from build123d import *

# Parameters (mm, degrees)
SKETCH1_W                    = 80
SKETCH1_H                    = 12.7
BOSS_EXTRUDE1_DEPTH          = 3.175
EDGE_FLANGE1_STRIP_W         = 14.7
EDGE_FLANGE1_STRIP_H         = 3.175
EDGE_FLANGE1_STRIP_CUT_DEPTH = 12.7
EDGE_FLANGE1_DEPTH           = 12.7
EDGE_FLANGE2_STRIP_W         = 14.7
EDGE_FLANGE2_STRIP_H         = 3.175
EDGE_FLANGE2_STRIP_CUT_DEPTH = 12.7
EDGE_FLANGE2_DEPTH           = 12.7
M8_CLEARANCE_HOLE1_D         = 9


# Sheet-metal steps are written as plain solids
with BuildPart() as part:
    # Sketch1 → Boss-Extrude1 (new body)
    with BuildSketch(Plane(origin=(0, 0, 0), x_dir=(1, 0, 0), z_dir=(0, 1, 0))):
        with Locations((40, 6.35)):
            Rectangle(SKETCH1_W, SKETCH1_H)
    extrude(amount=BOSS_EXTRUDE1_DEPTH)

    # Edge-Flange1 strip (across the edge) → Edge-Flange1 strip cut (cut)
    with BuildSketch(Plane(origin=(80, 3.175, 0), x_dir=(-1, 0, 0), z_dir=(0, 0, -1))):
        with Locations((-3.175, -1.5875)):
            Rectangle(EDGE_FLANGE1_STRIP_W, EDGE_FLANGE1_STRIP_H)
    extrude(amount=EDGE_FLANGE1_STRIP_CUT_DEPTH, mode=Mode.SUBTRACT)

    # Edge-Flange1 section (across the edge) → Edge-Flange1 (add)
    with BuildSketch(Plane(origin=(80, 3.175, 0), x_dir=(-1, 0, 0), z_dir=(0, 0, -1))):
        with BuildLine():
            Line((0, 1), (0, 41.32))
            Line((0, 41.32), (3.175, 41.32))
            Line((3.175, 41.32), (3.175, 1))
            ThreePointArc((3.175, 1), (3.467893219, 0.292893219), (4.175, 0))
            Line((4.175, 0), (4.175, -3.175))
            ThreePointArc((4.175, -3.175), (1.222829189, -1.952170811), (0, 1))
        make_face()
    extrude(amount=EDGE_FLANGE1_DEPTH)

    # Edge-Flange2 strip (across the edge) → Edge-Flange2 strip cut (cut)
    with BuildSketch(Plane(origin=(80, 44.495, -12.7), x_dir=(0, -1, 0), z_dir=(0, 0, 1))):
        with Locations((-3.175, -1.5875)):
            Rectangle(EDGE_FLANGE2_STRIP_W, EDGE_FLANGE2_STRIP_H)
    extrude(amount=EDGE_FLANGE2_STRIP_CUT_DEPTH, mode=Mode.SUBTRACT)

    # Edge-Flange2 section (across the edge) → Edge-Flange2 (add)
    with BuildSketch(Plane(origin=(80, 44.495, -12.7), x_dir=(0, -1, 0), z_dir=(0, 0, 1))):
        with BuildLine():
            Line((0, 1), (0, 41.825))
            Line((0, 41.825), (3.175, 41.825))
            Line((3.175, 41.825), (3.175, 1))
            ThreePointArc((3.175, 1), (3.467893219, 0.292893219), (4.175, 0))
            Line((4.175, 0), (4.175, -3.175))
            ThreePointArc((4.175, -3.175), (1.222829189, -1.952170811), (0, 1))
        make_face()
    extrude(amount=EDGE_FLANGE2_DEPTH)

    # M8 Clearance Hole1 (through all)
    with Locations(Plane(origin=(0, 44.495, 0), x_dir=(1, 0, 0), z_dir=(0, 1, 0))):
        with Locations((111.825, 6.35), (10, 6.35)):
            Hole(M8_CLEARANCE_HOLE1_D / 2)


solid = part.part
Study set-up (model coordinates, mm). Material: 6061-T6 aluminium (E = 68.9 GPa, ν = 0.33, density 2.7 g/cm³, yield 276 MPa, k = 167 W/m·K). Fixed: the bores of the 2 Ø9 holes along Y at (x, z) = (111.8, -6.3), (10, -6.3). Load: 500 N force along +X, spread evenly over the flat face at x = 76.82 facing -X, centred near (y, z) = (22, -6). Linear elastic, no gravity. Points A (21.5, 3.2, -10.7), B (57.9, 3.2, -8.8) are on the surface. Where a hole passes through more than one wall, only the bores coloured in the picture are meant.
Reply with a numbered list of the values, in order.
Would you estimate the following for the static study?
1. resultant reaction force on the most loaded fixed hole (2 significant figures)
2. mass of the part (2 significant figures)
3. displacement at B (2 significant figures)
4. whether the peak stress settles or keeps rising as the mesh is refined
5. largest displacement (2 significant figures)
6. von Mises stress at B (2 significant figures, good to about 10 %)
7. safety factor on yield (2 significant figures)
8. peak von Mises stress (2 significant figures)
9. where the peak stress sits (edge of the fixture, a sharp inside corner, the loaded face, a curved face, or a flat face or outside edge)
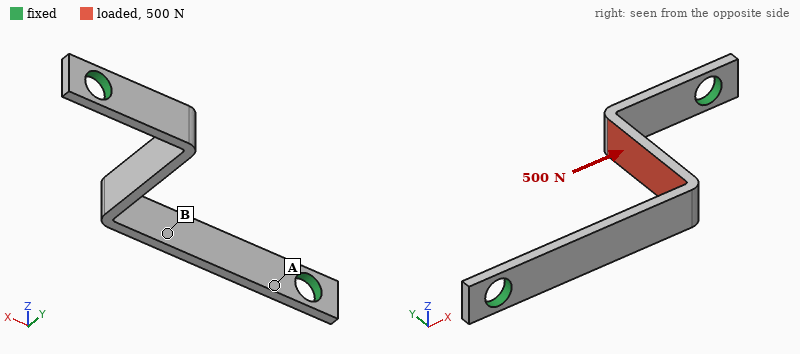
1. 260 N
2. 16 g
3. 0.039 mm
4. settles
5. 0.24 mm
6. 33 MPa
7. 2.7
8. 100 MPa
9. a flat face or outside edge
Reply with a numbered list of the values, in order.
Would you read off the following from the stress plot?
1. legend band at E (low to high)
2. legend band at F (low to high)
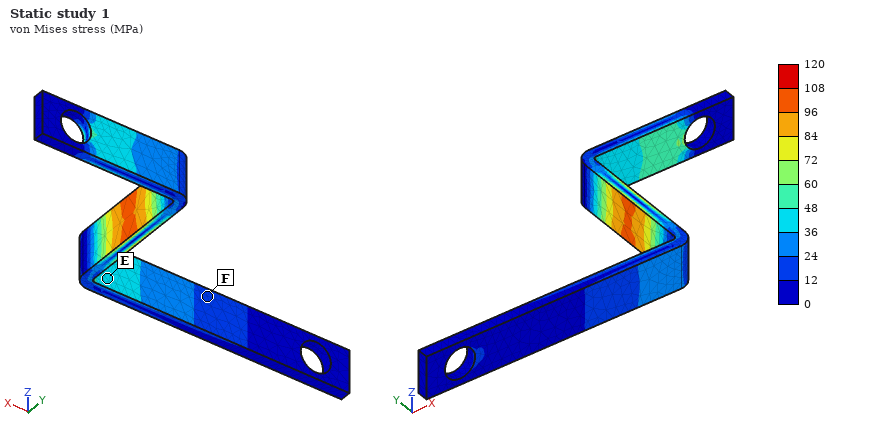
1. 36 to 48 MPa
2. 12 to 24 MPa
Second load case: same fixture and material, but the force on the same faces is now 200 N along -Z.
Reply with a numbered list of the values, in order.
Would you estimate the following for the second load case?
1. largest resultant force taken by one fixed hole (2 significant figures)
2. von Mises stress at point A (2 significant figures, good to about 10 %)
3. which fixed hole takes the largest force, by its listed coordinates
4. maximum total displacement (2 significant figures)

1. 120 N
2. 35 MPa
3. (111.8, -6.3)
4. 0.20 mm
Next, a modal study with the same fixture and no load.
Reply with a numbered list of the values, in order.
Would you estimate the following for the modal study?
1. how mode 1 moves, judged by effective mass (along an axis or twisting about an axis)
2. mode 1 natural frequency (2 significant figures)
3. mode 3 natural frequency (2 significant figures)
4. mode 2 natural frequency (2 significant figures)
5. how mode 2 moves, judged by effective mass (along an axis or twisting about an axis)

1. along Y
2. 1400 Hz
3. 3400 Hz
4. 1900 Hz
5. along Z
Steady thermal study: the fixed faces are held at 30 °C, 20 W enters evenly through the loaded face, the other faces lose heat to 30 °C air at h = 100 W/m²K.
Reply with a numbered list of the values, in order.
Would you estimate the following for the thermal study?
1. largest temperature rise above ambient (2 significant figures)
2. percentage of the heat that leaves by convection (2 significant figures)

1. 52 K
2. 46 %
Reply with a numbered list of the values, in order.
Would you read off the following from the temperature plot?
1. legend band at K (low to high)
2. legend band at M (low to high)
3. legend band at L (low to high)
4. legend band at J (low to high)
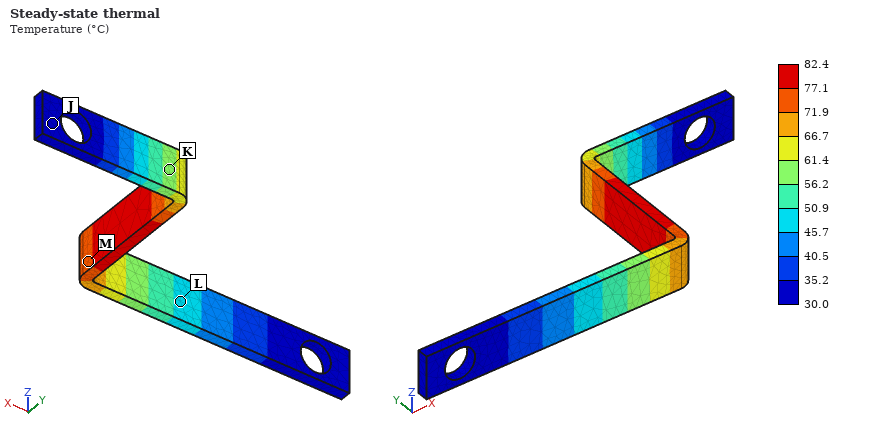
1. 56.2 to 61.4 °C
2. 71.9 to 77.1 °C
3. 45.7 to 50.9 °C
4. 30.0 to 35.2 °C
